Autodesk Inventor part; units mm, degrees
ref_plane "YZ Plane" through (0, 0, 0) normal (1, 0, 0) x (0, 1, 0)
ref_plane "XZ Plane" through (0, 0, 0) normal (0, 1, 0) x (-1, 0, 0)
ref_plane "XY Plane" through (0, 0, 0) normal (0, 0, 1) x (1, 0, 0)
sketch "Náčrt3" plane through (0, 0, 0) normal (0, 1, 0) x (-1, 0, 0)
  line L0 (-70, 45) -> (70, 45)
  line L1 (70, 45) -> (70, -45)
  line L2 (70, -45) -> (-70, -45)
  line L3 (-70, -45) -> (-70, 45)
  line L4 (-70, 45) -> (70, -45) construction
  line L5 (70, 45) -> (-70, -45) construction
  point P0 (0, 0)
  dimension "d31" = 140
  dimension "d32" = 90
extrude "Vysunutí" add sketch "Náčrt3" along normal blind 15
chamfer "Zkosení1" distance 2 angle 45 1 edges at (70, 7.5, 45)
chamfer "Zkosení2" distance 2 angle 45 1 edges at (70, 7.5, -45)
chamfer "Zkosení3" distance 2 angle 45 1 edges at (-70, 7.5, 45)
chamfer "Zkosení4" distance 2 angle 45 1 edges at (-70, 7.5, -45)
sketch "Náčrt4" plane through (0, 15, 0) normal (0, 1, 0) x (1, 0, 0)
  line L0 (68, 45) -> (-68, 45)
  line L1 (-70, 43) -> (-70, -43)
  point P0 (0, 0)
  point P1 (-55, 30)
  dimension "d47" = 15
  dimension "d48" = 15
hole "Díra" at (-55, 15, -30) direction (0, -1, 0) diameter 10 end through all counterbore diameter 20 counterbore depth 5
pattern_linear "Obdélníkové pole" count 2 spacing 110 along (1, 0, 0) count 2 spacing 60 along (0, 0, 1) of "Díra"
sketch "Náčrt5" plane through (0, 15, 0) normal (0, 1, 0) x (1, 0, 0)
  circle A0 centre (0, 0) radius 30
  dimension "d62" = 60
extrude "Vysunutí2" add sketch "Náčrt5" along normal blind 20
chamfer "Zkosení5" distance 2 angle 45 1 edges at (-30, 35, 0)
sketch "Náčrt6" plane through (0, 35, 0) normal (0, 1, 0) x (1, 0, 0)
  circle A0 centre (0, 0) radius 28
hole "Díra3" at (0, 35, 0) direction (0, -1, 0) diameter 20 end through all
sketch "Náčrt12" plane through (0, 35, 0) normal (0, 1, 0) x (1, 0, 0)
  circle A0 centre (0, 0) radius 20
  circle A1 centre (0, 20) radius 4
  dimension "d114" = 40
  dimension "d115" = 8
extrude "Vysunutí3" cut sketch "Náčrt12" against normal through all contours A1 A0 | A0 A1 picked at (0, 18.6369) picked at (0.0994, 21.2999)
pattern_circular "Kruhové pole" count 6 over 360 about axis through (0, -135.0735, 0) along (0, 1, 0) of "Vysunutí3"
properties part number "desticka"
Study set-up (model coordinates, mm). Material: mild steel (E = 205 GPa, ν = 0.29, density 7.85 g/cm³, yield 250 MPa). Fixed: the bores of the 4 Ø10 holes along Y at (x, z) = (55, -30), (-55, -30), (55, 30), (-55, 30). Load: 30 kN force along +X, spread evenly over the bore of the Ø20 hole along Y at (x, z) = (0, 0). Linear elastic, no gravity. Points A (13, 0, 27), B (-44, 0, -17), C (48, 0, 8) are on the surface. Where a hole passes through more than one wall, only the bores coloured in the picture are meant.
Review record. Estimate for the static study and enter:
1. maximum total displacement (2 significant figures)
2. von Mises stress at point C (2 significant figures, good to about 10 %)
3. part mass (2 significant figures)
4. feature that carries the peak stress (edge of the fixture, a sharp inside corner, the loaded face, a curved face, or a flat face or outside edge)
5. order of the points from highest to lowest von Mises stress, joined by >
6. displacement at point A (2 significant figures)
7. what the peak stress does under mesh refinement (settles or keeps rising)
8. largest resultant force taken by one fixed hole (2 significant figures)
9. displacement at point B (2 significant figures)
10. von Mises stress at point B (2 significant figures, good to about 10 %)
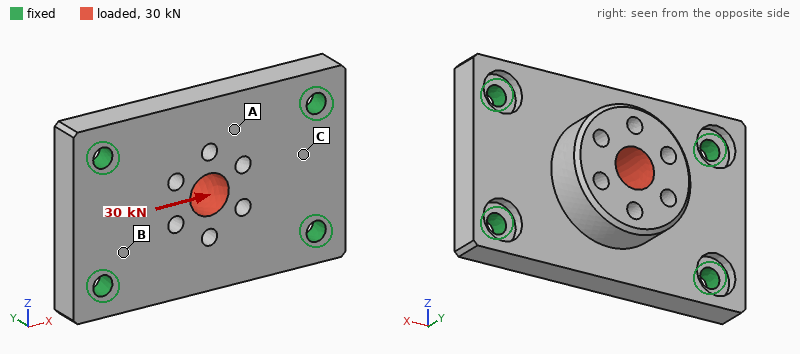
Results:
9.8 µm
9.7 MPa
1.7 kg
edge of the fixture
B > C > A
2.5 µm
keeps rising
8.0 kN
2.8 µm
18 MPa
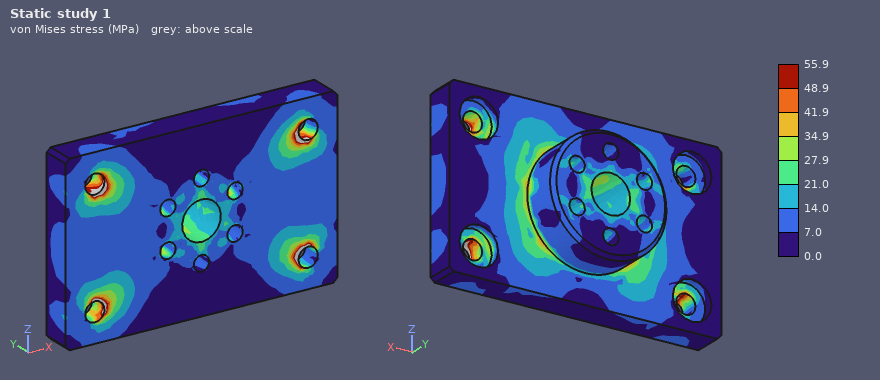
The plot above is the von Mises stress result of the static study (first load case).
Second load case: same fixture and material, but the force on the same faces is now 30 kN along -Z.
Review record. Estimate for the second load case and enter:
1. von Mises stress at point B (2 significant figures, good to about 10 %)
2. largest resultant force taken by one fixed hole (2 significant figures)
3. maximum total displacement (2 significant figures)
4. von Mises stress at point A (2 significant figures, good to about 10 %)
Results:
18 MPa
10 kN
21 µm
17 MPa
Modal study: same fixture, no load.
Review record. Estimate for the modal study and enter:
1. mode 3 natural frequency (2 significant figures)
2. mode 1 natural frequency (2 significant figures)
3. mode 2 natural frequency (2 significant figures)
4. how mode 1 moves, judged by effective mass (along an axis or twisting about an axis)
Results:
9900 Hz
4800 Hz
5800 Hz
along Y
